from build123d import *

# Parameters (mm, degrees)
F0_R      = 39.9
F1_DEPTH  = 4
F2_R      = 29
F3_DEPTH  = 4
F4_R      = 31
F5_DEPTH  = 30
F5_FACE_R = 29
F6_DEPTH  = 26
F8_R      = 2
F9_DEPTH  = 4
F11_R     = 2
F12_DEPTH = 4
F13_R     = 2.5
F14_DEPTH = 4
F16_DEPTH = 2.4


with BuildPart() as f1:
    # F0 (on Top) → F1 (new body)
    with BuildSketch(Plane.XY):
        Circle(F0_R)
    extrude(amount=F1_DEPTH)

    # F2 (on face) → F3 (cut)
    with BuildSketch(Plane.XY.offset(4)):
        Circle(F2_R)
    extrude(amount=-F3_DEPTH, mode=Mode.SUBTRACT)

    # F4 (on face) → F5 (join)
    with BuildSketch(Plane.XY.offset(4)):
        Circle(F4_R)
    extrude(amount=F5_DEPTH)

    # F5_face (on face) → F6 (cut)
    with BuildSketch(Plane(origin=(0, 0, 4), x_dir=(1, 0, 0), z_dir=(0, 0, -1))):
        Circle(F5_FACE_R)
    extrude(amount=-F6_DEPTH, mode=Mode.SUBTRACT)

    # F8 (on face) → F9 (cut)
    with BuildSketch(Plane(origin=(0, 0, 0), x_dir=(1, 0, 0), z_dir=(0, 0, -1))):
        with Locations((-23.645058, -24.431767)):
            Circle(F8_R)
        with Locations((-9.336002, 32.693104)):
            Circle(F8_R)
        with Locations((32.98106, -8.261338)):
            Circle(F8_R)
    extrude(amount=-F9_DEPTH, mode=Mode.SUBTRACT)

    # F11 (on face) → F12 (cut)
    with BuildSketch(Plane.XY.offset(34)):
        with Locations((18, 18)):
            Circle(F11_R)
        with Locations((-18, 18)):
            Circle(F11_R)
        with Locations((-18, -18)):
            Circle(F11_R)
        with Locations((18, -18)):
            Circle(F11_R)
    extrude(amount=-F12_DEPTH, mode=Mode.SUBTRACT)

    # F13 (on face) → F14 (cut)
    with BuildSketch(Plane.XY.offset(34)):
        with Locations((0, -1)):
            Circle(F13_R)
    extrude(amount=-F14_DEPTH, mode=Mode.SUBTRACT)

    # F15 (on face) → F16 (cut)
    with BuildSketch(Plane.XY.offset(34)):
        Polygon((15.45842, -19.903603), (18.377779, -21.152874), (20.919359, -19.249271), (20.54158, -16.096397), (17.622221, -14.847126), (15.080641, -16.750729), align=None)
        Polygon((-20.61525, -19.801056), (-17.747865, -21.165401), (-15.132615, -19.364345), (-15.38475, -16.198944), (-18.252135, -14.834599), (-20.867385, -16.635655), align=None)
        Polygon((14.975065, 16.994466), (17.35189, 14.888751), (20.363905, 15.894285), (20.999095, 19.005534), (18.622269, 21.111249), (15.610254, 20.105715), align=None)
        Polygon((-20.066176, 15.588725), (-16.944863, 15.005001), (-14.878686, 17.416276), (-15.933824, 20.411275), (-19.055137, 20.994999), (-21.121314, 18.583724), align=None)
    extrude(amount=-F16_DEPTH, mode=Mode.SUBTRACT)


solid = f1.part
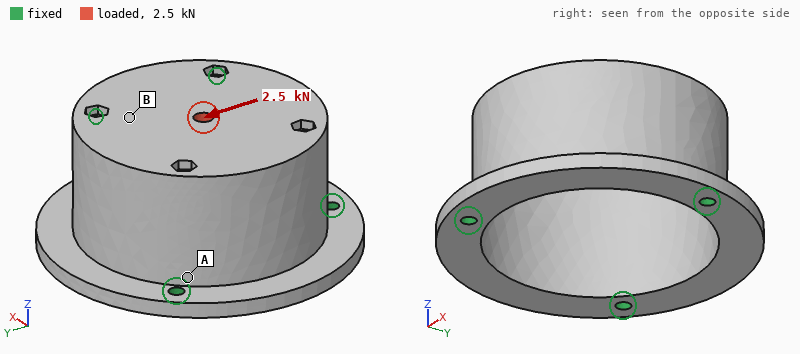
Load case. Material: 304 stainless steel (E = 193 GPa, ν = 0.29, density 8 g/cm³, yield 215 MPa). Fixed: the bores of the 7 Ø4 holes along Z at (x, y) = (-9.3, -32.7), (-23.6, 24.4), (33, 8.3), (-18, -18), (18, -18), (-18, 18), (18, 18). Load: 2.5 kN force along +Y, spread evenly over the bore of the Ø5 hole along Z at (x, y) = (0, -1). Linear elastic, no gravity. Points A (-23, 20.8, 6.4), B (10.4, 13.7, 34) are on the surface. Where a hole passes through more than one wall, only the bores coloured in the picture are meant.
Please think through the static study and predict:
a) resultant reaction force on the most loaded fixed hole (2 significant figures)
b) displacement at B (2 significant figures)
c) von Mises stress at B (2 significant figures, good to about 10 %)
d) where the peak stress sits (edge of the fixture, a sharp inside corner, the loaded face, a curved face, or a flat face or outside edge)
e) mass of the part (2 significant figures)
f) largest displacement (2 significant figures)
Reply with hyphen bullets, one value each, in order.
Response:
- 640 N
- 1.2 µm
- 9.8 MPa
- edge of the fixture
- 250 g
- 2.9 µm
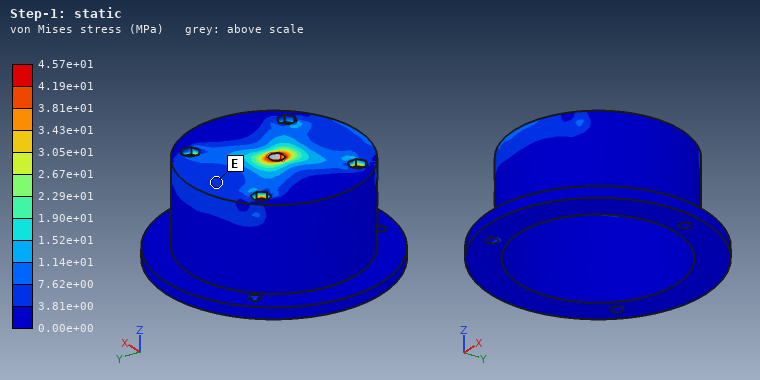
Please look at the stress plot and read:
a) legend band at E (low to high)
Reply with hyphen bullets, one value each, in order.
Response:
- 3.81e+00 to 7.62e+00 MPa
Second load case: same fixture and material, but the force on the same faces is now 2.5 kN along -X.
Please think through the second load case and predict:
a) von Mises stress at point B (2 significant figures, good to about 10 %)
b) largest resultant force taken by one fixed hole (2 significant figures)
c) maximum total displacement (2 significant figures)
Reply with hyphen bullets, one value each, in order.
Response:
- 8.9 MPa
- 660 N
- 2.9 µm
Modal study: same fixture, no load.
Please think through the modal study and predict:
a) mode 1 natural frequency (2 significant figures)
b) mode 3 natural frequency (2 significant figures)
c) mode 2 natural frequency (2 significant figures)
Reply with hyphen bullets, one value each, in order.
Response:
- 9800 Hz
- 11 kHz
- 11 kHz
